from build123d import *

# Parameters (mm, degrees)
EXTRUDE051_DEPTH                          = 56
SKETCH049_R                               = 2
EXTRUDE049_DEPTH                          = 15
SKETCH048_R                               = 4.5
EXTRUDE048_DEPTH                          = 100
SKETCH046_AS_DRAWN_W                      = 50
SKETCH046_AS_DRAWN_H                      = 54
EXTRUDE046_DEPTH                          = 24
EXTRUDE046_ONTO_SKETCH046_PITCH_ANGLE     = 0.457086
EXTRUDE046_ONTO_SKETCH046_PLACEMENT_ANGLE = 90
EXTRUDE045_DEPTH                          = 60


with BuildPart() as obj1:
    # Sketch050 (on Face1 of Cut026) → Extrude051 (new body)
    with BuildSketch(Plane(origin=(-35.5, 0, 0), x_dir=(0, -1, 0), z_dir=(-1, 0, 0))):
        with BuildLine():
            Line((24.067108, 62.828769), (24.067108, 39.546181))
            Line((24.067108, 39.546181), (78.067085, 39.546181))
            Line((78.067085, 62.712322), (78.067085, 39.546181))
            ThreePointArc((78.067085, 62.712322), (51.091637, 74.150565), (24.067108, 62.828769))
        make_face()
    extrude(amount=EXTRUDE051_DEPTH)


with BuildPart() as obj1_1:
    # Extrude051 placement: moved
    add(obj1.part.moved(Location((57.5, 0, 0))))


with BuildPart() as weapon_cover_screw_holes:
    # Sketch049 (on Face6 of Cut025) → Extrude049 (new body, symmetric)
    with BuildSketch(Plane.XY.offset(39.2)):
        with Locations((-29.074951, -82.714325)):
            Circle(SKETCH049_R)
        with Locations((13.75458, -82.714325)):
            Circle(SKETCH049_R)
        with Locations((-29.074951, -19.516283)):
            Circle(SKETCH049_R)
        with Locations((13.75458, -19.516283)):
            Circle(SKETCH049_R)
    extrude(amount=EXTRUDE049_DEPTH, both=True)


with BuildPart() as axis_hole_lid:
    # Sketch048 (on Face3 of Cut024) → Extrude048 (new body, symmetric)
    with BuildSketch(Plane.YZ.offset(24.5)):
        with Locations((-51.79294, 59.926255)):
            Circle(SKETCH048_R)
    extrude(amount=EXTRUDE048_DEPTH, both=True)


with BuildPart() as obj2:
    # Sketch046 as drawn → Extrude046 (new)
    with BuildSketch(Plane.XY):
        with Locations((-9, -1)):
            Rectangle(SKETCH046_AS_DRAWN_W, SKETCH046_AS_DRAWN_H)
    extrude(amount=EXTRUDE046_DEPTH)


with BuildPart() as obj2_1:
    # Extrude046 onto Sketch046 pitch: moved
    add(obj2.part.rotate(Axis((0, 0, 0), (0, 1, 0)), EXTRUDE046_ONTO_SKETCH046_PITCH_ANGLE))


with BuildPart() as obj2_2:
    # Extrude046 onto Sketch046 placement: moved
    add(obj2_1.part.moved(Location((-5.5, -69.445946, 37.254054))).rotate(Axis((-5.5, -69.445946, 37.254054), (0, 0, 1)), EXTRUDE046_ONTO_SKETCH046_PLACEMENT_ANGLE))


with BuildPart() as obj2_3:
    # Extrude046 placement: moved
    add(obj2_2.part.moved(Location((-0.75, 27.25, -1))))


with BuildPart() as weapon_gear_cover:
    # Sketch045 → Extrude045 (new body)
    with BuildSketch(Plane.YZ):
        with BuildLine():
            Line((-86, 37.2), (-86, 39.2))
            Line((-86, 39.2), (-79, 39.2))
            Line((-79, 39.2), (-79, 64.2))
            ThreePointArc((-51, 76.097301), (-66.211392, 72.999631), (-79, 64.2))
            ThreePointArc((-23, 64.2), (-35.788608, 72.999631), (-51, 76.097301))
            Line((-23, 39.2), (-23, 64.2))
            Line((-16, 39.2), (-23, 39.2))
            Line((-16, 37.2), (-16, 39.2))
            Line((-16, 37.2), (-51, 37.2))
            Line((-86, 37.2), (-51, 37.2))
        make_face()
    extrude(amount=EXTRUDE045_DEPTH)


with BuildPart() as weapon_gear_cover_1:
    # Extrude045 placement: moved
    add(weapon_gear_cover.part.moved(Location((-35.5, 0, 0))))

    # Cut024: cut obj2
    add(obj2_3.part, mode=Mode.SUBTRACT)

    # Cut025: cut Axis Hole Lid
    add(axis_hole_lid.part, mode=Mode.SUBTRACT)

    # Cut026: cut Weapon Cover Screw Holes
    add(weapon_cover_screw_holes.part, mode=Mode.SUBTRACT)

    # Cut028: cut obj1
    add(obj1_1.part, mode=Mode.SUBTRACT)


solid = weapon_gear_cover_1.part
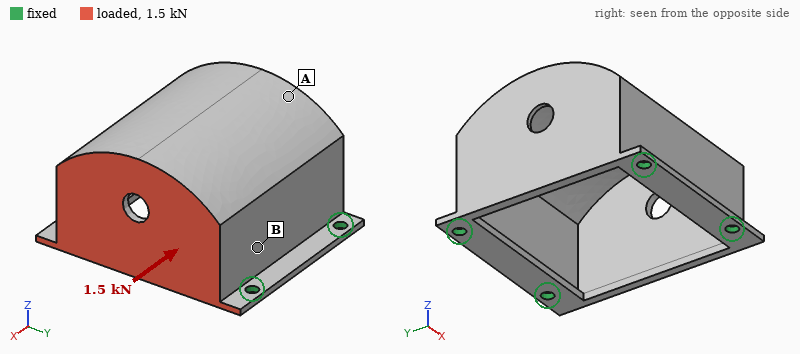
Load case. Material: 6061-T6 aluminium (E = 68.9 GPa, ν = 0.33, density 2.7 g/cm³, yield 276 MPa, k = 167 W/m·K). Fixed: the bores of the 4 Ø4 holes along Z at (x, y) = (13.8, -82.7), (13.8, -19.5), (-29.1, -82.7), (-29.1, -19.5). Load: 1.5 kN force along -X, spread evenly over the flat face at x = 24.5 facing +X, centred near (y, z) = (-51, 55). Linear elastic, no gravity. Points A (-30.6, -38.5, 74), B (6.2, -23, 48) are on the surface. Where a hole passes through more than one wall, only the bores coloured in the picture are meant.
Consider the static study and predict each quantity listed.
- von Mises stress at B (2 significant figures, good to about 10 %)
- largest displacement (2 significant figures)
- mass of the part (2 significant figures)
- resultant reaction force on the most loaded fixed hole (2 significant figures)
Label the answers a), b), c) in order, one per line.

a) 28 MPa
b) 0.25 mm
c) 52 g
d) 630 N
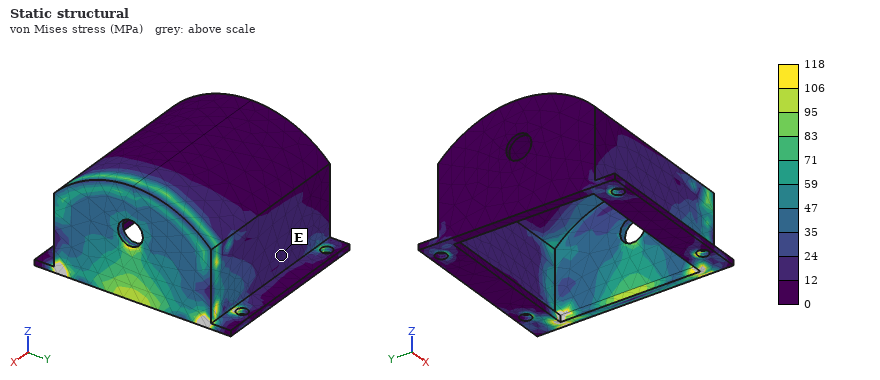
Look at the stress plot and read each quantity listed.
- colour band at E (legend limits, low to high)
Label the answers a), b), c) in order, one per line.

a) 12 to 24 MPa
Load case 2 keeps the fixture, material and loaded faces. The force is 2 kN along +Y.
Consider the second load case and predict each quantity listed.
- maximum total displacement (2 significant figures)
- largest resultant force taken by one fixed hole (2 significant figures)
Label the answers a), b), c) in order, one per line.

a) 57 µm
b) 1.0 kN
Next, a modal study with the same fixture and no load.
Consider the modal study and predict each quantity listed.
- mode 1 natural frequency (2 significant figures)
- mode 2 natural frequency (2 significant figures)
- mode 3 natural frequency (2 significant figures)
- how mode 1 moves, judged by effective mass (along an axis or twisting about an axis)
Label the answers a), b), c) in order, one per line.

a) 4000 Hz
b) 4300 Hz
c) 5100 Hz
d) along X
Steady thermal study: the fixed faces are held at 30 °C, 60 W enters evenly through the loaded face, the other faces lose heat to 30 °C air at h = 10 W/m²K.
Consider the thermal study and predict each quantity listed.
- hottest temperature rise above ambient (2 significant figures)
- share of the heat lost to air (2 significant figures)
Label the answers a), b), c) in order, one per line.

a) 74 K
b) 11 %
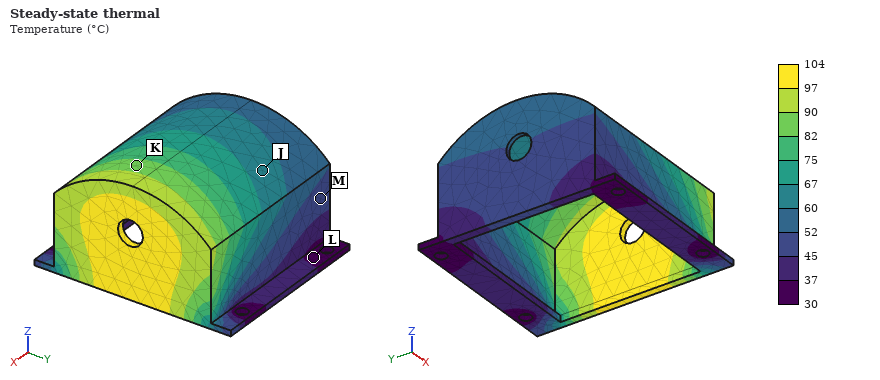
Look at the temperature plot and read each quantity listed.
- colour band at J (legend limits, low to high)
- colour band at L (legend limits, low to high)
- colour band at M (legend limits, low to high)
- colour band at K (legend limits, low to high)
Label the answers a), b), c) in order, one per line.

a) 60 to 67 °C
b) 30 to 37 °C
c) 45 to 52 °C
d) 82 to 90 °C
